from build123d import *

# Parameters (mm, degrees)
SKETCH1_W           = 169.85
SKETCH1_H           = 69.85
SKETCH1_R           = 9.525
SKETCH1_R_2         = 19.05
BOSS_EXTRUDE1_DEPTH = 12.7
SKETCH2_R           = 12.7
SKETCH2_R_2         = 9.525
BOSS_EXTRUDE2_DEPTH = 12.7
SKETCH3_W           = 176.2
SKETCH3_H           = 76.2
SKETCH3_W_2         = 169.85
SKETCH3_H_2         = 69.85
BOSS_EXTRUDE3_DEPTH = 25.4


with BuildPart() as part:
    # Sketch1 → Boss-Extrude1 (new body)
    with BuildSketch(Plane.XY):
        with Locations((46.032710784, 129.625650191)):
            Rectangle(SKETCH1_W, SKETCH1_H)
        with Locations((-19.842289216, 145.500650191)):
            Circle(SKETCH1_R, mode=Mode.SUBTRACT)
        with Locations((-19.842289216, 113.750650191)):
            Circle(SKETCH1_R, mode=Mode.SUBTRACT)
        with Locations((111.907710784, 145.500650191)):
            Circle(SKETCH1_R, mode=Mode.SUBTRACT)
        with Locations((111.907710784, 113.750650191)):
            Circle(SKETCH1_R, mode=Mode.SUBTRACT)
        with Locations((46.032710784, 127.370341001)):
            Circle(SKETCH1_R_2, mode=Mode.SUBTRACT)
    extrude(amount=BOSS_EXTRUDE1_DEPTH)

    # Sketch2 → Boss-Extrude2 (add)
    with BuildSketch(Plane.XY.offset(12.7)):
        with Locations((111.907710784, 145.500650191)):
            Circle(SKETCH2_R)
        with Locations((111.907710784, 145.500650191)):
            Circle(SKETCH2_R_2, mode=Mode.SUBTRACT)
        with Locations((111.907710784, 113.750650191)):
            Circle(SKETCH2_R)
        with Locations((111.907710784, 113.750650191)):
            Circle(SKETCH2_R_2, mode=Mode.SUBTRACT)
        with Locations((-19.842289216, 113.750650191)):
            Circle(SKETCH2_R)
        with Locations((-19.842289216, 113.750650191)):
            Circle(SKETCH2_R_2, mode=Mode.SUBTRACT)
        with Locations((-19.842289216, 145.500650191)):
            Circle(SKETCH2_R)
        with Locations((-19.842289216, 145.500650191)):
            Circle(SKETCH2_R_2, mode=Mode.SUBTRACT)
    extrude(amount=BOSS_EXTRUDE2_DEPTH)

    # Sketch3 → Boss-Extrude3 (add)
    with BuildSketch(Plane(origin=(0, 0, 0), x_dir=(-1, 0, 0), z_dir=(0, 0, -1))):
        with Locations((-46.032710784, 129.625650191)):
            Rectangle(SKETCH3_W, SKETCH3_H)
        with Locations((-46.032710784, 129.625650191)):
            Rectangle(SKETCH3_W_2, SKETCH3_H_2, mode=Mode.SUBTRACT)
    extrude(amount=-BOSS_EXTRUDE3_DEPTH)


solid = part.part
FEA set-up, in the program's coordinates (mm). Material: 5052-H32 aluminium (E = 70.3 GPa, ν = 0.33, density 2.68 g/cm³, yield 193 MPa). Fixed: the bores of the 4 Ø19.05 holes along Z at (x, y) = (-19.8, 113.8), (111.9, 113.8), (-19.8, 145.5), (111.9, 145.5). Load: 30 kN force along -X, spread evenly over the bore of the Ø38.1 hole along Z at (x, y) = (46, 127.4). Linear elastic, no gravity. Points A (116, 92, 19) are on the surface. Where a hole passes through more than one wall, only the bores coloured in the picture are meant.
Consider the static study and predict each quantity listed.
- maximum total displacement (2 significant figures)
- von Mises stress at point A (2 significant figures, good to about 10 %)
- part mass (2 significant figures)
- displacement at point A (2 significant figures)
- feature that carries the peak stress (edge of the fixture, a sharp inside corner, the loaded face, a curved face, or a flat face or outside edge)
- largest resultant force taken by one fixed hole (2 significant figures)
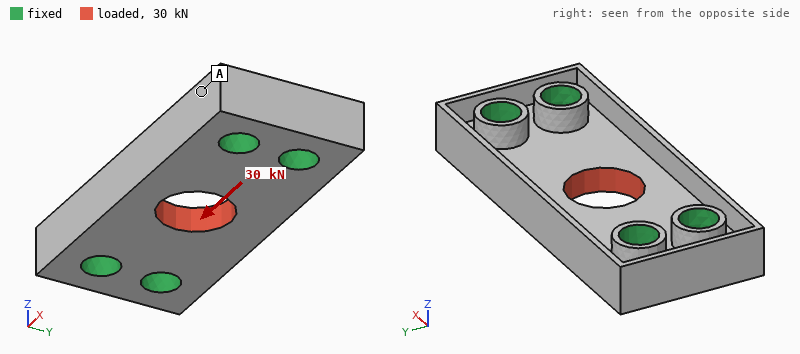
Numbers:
15 µm
4.0 MPa
460 g
3.6 µm
the loaded face
8.0 kN
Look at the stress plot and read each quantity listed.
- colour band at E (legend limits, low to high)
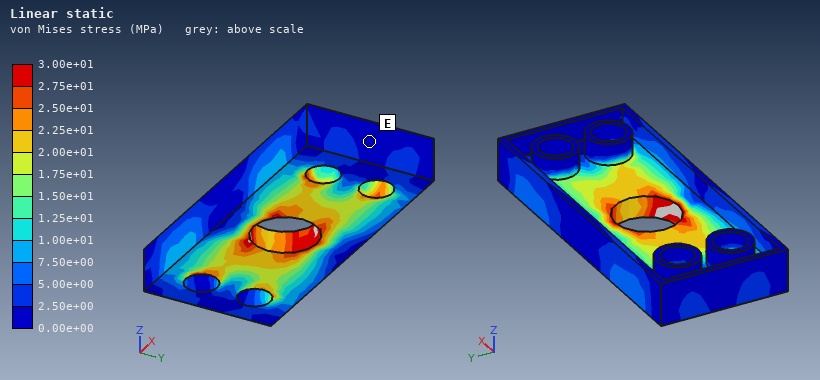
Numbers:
0.00e+00 to 2.50e+00 MPa
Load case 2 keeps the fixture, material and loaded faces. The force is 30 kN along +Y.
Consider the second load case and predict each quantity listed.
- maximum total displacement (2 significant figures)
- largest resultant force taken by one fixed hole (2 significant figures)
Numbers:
56 µm
10 kN
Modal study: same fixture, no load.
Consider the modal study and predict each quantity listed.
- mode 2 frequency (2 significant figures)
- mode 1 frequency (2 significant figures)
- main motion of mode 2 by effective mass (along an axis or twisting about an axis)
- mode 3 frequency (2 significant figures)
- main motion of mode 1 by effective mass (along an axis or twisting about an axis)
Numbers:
6000 Hz
5500 Hz
twisting about X
10 kHz
along Z
